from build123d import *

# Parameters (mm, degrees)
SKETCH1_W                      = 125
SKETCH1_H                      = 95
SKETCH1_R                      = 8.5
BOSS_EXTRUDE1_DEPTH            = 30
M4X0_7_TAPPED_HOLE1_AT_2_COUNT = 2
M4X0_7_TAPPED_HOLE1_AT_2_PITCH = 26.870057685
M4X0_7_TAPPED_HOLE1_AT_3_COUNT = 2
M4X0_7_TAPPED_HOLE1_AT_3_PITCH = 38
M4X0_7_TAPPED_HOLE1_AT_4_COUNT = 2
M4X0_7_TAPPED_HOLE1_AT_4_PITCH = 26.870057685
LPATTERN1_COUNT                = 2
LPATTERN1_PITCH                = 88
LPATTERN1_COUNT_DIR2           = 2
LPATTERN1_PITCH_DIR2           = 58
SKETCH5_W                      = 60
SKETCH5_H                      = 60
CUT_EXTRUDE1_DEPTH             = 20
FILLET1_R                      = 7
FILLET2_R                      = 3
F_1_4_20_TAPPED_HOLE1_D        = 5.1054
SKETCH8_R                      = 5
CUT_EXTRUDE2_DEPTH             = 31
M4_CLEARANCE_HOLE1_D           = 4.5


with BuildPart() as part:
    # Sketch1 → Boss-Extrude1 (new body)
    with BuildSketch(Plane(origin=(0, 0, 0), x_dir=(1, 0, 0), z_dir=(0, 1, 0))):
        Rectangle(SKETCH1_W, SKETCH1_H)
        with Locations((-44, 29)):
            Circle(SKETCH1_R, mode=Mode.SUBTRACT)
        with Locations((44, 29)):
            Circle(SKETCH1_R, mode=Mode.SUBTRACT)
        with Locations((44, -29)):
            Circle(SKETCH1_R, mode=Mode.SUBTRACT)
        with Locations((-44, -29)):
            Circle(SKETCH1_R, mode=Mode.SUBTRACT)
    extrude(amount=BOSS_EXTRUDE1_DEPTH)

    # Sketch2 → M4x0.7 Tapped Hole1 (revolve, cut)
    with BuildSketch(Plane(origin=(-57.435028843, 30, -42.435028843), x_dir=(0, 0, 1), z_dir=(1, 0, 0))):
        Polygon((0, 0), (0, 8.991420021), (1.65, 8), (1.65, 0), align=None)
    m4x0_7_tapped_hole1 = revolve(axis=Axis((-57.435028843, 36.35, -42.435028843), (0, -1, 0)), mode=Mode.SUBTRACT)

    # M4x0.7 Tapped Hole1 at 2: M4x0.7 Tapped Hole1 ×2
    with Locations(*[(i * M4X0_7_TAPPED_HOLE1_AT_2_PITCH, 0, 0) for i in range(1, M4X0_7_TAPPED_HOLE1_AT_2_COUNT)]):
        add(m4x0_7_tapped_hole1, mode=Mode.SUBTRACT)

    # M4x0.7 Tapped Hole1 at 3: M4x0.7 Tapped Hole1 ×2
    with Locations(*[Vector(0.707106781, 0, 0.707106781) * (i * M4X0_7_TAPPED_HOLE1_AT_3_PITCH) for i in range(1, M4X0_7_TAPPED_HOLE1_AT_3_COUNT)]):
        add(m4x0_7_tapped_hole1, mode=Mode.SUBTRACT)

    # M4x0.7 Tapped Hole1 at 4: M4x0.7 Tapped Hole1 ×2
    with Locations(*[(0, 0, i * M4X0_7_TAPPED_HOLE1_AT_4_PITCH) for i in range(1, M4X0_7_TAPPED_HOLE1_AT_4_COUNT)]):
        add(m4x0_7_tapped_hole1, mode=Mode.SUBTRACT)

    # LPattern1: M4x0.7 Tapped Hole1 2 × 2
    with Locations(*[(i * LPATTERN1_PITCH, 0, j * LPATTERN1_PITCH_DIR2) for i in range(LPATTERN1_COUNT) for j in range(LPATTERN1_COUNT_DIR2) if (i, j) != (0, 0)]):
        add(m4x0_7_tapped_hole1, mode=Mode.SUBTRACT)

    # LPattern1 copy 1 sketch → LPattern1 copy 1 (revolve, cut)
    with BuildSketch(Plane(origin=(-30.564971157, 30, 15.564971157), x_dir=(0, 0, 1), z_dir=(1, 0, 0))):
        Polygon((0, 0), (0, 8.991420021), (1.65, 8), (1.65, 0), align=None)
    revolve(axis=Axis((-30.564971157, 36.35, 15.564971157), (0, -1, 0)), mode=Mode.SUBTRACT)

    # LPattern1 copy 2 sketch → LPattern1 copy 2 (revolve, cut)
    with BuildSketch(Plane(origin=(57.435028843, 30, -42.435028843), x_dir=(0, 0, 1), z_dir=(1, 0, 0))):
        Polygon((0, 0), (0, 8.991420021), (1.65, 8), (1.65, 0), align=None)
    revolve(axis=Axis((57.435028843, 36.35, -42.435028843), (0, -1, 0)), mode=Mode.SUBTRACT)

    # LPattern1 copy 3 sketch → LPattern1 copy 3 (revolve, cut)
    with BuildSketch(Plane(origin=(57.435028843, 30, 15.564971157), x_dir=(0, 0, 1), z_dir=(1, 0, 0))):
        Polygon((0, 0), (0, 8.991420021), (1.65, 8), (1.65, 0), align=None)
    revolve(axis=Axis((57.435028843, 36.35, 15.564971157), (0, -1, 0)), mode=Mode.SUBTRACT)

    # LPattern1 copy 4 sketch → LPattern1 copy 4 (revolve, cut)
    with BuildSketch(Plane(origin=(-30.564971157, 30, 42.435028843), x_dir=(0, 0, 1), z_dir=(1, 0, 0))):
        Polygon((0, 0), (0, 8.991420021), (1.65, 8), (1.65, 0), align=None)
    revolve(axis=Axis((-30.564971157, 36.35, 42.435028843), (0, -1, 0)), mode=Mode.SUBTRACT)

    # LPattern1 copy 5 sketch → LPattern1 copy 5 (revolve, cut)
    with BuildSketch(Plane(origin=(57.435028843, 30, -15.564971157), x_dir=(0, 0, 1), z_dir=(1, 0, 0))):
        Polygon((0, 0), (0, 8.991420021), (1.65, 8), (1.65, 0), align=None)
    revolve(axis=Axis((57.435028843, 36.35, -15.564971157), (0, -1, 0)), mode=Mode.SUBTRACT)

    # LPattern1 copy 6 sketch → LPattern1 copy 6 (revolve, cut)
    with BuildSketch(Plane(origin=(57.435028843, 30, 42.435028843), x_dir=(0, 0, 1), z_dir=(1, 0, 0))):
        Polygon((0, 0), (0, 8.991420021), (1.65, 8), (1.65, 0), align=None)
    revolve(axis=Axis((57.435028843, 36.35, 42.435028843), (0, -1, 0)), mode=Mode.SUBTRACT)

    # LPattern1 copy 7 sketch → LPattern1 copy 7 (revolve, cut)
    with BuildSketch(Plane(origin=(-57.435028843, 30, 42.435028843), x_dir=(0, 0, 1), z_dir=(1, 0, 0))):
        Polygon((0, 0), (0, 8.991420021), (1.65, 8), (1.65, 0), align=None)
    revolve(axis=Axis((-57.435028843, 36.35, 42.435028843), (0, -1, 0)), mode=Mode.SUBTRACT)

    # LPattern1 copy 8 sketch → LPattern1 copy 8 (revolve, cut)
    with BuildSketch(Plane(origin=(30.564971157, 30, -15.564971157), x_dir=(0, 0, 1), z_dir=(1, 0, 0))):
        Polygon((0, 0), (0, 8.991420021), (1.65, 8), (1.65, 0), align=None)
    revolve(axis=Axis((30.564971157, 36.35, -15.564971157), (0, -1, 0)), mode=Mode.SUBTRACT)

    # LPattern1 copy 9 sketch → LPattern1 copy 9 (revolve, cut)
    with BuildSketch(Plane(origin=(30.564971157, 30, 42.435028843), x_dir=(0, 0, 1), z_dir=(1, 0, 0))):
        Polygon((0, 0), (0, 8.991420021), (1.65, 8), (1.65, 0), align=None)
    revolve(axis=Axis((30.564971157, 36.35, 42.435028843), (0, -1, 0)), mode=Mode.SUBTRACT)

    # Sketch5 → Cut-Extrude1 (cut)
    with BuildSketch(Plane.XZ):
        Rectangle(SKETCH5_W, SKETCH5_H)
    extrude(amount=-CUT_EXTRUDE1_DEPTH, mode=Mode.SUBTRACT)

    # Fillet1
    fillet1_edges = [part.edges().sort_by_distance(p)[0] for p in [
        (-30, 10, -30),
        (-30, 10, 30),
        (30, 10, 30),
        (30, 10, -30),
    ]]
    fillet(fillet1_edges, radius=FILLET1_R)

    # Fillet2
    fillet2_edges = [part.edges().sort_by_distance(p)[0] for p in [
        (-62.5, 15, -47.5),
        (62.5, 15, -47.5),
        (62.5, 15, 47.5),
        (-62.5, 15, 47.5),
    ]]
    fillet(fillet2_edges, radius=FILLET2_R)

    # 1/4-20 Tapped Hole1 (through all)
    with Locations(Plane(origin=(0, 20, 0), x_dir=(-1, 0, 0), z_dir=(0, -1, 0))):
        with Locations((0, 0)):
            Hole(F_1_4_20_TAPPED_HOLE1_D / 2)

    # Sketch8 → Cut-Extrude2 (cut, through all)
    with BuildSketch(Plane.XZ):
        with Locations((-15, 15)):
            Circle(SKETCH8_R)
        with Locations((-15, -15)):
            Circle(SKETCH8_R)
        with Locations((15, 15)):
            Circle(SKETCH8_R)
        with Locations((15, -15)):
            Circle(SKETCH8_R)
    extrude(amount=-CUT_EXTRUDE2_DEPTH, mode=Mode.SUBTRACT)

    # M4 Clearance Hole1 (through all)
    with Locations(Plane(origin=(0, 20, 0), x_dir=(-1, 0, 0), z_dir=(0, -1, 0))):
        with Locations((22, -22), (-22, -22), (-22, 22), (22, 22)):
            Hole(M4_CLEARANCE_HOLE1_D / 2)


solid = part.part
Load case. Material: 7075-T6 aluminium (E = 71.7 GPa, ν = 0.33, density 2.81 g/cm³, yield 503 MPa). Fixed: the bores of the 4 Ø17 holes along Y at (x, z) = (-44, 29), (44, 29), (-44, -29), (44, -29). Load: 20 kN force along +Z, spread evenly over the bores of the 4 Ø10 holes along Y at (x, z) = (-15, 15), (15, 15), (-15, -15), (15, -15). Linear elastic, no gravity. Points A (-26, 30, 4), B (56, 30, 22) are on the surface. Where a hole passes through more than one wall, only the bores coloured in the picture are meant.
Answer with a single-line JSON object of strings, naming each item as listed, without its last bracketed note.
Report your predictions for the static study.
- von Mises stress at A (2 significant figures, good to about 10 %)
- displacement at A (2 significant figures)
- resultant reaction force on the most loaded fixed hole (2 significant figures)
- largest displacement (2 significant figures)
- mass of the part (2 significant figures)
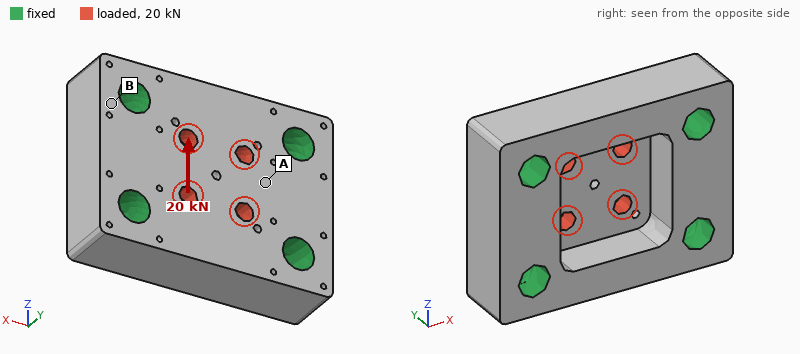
{"von Mises stress at A": "17 MPa", "displacement at A": "4.8 µm", "resultant reaction force on the most loaded fixed hole": "5.4 kN", "largest displacement": "13 µm", "mass of the part": "710 g"}
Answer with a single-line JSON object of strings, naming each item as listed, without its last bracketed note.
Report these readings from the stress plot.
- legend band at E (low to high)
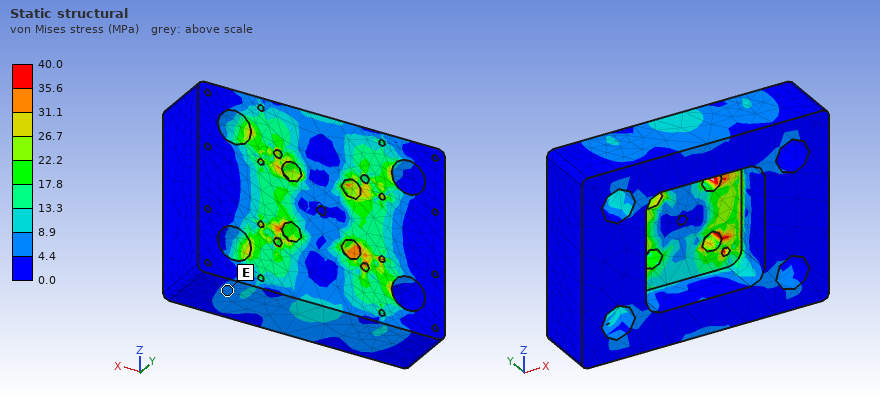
{"legend band at E": "4.4 to 8.9 MPa"}
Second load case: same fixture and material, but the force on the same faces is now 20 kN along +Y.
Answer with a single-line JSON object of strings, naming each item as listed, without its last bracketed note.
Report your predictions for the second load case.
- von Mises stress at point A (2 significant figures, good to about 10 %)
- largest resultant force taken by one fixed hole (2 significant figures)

{"von Mises stress at point A": "26 MPa", "largest resultant force taken by one fixed hole": "5.3 kN"}
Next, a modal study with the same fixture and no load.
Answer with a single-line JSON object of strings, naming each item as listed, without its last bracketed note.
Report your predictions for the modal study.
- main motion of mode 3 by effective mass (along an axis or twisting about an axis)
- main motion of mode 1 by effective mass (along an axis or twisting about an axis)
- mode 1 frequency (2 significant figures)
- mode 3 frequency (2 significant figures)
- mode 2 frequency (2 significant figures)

{"main motion of mode 3 by effective mass": "along Z", "main motion of mode 1 by effective mass": "along Y", "mode 1 frequency": "12 kHz", "mode 3 frequency": "16 kHz", "mode 2 frequency": "15 kHz"}
